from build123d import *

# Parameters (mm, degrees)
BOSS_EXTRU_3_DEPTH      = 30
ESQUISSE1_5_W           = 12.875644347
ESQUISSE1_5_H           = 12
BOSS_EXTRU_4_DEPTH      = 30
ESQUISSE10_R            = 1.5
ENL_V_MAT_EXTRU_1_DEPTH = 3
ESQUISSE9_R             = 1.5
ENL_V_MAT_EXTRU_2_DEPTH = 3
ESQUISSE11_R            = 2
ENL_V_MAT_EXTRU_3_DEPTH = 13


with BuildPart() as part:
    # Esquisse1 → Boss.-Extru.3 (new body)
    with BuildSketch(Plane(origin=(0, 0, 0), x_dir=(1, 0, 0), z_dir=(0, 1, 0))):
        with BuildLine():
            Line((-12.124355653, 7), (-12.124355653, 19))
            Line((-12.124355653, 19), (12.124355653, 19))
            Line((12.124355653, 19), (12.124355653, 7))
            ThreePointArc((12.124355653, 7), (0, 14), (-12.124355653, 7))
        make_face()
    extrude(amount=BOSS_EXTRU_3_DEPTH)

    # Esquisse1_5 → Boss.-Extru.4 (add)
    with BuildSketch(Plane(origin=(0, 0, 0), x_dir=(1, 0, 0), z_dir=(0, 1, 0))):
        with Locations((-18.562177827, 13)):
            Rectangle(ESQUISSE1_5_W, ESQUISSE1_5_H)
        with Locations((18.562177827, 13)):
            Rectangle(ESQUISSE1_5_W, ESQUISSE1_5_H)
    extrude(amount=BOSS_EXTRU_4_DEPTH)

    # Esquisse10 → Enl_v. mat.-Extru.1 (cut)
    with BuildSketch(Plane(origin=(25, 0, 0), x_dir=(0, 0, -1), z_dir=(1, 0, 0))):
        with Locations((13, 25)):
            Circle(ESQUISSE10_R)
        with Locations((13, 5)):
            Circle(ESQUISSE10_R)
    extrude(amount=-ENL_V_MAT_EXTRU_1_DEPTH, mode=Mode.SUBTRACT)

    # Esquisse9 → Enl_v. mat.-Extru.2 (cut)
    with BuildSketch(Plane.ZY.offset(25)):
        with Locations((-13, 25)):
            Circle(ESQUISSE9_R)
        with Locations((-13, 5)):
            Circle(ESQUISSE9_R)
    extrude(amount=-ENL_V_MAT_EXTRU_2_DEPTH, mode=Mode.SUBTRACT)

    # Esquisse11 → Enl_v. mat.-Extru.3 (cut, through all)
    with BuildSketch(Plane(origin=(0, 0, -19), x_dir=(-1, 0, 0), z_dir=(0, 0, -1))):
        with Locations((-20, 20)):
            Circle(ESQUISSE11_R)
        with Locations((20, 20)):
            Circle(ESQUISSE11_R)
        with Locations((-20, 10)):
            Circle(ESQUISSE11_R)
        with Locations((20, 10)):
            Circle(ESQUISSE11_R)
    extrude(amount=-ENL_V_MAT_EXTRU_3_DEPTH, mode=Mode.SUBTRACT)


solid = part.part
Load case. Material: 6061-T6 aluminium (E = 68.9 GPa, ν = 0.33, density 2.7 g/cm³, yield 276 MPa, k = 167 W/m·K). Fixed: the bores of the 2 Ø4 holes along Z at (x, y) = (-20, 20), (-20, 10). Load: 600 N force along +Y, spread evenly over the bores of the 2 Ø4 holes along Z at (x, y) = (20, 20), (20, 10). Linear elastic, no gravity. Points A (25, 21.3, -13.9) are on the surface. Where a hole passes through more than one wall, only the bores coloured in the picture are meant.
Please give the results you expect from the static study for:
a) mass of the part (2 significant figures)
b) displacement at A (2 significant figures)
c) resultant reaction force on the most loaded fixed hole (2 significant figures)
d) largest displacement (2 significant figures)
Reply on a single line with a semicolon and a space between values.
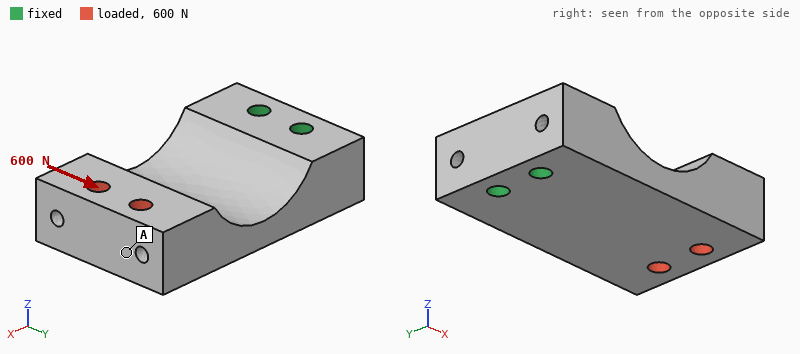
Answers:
37 g; 30 µm; 1.7 kN; 36 µm
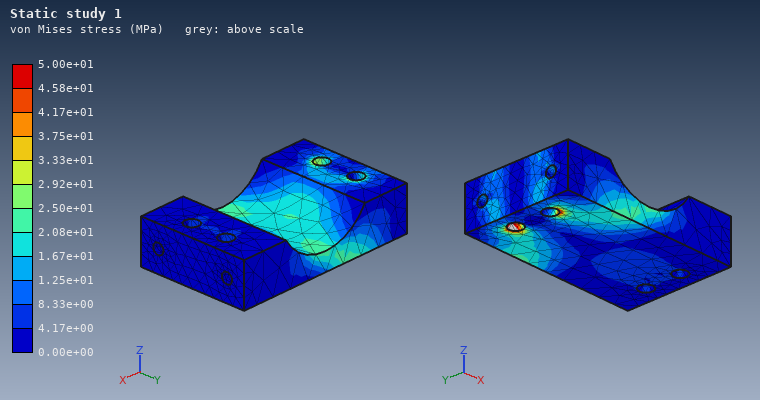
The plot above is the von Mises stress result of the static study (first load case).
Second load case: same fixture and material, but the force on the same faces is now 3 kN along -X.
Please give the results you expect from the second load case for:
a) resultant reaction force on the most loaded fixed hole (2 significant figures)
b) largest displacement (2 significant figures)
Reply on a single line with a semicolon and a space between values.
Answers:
1.5 kN; 0.15 mm
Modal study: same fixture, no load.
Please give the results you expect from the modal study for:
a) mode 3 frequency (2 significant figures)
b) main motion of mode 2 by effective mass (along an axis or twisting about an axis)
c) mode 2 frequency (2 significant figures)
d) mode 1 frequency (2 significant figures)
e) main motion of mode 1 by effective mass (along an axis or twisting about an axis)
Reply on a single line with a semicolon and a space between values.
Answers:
8200 Hz; along Y; 6000 Hz; 2600 Hz; along Z
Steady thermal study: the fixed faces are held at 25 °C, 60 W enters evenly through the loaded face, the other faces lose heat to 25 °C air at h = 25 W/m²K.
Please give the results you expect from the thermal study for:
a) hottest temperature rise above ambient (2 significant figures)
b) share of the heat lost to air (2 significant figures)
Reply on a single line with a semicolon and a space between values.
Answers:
65 K; 6.2 %
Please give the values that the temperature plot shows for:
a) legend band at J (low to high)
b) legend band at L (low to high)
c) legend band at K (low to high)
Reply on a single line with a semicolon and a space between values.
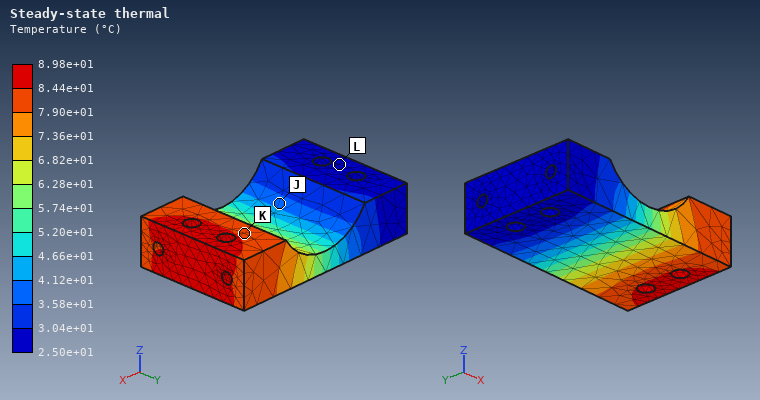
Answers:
3.58e+01 to 4.12e+01 °C; 2.50e+01 to 3.04e+01 °C; 7.90e+01 to 8.44e+01 °C
